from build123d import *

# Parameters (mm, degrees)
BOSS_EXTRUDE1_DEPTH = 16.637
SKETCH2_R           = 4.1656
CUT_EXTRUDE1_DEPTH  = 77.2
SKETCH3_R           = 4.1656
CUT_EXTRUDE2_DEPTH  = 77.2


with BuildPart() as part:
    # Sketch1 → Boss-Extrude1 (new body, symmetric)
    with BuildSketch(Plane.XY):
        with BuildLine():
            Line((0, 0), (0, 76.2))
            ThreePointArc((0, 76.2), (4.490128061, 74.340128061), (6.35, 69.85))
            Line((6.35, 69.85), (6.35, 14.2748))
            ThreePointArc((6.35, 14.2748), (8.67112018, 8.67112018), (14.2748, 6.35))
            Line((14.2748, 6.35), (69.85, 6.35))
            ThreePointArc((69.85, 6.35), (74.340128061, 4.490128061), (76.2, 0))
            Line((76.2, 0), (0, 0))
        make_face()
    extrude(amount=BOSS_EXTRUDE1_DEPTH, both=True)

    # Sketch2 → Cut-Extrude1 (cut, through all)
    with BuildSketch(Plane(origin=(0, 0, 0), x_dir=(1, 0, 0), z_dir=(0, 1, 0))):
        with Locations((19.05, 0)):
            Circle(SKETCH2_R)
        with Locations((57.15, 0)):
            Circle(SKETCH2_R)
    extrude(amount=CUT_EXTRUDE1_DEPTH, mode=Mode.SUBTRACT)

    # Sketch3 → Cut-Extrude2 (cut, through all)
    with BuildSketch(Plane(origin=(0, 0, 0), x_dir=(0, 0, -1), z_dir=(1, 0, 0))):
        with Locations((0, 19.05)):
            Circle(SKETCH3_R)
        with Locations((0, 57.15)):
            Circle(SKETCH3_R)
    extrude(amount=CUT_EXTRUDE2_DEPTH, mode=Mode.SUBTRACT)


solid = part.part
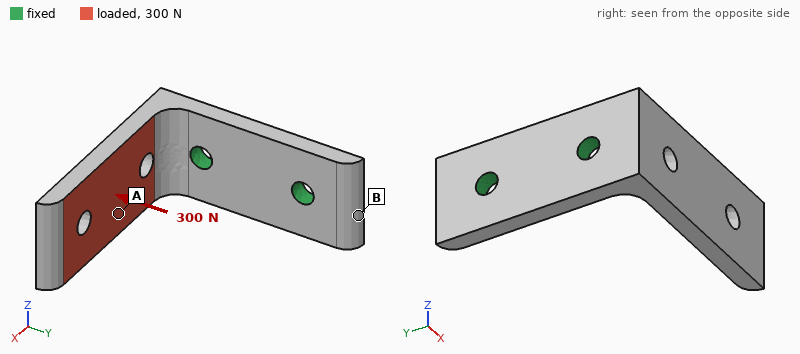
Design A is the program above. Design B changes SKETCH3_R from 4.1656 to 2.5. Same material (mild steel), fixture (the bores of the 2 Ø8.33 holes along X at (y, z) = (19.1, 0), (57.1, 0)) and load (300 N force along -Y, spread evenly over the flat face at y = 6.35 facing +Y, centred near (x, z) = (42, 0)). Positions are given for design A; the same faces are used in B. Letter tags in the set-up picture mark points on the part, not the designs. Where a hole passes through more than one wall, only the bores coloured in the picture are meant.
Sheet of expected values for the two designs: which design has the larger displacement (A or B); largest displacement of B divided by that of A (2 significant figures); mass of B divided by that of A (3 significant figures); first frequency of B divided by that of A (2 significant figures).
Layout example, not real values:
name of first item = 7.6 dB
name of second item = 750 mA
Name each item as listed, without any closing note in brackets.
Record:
which design has the larger displacement = B
largest displacement of B divided by that of A = 1.1
mass of B divided by that of A = 1.02
first frequency of B divided by that of A = 0.95
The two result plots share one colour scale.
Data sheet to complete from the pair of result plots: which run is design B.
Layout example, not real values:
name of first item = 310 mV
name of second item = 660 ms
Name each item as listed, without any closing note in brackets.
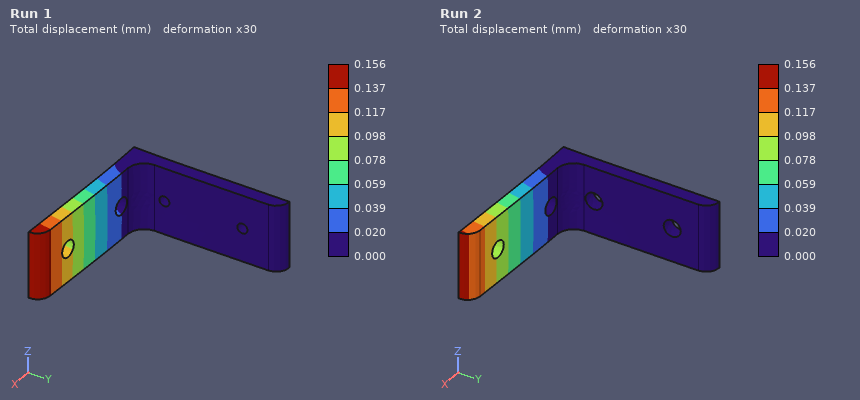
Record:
which run is design B = Run 1
